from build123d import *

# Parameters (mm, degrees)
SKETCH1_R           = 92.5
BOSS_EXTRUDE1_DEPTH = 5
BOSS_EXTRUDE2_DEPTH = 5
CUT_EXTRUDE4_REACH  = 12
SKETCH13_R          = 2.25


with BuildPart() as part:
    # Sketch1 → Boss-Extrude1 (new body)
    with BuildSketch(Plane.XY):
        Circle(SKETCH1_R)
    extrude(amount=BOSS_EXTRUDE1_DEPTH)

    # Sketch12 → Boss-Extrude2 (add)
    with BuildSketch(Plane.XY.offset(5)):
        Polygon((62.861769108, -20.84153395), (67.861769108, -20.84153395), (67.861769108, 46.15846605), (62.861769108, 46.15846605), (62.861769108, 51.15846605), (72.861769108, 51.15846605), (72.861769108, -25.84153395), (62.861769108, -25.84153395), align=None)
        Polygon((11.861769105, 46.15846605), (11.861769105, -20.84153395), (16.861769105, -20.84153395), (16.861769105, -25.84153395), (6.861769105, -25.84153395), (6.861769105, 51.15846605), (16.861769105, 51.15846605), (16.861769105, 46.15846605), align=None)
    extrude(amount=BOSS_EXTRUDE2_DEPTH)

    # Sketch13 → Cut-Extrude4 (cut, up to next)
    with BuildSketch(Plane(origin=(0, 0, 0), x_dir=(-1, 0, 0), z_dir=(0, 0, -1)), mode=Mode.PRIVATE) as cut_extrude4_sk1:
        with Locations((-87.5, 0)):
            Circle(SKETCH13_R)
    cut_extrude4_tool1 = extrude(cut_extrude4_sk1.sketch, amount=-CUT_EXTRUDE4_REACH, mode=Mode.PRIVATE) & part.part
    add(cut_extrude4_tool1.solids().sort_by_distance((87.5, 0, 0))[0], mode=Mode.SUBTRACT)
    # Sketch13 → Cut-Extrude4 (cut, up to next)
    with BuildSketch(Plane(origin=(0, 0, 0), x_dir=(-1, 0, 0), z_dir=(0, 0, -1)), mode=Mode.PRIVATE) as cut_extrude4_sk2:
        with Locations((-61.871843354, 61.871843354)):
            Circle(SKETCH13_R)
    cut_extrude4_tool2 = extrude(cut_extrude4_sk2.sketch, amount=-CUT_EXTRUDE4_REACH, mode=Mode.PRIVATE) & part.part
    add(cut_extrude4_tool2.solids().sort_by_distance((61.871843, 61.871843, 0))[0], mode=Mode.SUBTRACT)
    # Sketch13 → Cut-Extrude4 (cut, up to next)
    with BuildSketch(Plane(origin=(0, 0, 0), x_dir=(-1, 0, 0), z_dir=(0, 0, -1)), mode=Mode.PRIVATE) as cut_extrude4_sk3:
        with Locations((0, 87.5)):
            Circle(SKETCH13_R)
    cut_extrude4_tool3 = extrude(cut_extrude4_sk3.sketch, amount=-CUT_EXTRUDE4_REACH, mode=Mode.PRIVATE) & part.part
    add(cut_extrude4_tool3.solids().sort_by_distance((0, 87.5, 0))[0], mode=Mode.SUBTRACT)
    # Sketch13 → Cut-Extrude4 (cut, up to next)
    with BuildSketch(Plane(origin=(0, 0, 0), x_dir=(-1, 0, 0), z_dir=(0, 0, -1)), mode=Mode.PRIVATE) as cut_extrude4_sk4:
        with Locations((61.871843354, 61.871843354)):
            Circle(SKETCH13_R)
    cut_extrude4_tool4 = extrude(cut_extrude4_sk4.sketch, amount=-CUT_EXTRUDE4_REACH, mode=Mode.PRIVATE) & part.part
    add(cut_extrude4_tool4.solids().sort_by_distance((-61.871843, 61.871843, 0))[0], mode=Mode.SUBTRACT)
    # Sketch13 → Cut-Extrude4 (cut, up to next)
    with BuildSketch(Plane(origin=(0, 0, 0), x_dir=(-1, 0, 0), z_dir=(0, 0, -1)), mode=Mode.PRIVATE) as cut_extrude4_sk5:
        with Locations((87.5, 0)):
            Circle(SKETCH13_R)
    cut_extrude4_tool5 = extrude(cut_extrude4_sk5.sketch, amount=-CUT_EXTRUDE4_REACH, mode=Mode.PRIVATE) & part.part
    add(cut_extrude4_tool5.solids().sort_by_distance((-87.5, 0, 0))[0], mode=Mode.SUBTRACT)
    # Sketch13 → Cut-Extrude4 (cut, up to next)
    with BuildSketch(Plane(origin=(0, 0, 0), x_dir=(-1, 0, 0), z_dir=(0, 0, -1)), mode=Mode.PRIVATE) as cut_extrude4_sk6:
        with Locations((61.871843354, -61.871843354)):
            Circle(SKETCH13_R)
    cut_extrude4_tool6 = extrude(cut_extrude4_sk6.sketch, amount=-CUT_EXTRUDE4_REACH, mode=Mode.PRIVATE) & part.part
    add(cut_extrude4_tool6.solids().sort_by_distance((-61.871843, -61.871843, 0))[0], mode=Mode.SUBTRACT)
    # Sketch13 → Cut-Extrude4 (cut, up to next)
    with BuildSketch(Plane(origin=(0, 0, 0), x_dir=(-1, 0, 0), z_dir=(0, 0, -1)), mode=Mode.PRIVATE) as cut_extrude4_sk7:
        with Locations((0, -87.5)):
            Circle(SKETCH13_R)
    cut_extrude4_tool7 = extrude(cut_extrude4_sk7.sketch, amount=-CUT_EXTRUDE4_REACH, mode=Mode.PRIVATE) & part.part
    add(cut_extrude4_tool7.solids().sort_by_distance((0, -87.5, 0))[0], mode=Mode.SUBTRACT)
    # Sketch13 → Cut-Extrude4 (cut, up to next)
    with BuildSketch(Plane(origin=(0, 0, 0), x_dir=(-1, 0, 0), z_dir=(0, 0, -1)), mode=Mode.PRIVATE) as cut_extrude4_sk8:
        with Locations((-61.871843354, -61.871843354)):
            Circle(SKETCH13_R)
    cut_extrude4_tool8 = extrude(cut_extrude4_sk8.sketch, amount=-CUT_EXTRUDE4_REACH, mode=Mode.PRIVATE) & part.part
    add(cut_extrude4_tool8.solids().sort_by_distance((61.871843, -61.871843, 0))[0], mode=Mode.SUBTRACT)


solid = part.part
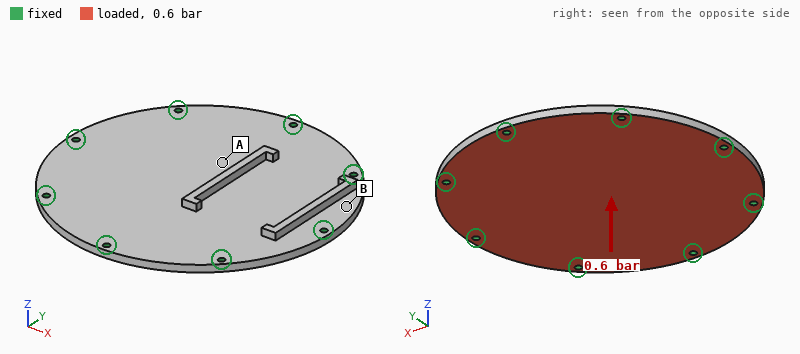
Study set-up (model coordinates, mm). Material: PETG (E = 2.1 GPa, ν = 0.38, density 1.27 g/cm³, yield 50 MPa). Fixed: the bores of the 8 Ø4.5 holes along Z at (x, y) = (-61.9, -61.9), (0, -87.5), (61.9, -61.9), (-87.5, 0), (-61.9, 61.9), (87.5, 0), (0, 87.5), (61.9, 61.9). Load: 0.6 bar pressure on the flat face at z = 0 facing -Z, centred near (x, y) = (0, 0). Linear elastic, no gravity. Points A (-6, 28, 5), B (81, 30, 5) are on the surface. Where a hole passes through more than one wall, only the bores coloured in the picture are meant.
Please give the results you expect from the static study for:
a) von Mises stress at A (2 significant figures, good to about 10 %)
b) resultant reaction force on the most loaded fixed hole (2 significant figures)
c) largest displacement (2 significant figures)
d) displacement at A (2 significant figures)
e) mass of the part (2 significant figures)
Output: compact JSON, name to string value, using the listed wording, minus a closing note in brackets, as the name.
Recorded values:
{"von Mises stress at A": "8.6 MPa", "resultant reaction force on the most loaded fixed hole": "210 N", "largest displacement": "2.9 mm", "displacement at A": "2.5 mm", "mass of the part": "180 g"}
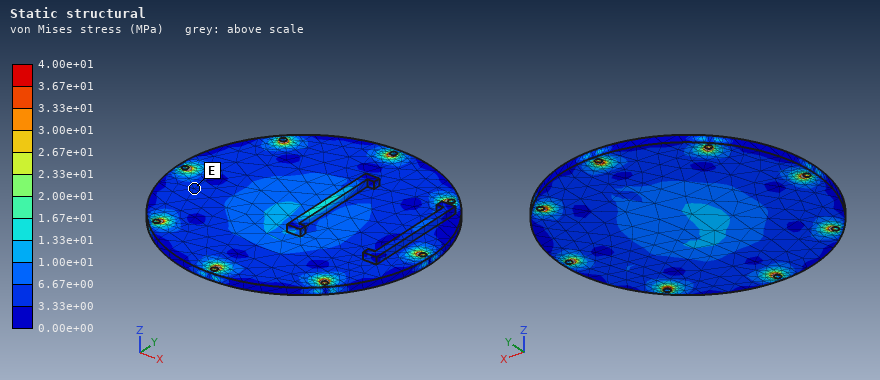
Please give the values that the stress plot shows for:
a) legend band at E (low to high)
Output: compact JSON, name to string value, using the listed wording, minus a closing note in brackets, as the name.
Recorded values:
{"legend band at E": "3.33e+00 to 6.67e+00 MPa"}
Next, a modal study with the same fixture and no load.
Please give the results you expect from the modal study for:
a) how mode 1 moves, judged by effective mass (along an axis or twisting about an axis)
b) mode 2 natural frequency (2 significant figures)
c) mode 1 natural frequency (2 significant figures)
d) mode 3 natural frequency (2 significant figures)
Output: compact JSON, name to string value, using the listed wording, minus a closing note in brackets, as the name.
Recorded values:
{"how mode 1 moves, judged by effective mass": "along Z", "mode 2 natural frequency": "730 Hz", "mode 1 natural frequency": "340 Hz", "mode 3 natural frequency": "750 Hz"}
